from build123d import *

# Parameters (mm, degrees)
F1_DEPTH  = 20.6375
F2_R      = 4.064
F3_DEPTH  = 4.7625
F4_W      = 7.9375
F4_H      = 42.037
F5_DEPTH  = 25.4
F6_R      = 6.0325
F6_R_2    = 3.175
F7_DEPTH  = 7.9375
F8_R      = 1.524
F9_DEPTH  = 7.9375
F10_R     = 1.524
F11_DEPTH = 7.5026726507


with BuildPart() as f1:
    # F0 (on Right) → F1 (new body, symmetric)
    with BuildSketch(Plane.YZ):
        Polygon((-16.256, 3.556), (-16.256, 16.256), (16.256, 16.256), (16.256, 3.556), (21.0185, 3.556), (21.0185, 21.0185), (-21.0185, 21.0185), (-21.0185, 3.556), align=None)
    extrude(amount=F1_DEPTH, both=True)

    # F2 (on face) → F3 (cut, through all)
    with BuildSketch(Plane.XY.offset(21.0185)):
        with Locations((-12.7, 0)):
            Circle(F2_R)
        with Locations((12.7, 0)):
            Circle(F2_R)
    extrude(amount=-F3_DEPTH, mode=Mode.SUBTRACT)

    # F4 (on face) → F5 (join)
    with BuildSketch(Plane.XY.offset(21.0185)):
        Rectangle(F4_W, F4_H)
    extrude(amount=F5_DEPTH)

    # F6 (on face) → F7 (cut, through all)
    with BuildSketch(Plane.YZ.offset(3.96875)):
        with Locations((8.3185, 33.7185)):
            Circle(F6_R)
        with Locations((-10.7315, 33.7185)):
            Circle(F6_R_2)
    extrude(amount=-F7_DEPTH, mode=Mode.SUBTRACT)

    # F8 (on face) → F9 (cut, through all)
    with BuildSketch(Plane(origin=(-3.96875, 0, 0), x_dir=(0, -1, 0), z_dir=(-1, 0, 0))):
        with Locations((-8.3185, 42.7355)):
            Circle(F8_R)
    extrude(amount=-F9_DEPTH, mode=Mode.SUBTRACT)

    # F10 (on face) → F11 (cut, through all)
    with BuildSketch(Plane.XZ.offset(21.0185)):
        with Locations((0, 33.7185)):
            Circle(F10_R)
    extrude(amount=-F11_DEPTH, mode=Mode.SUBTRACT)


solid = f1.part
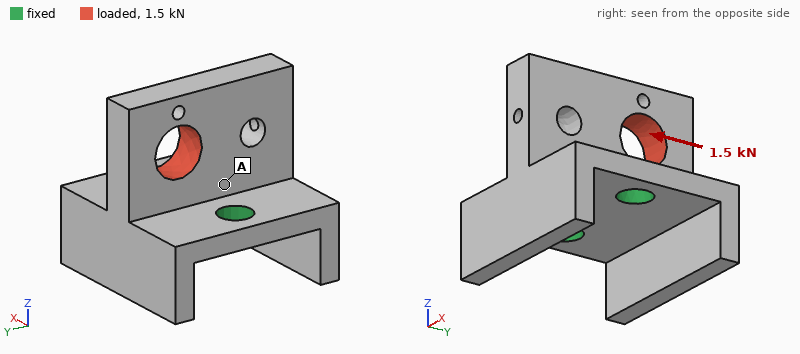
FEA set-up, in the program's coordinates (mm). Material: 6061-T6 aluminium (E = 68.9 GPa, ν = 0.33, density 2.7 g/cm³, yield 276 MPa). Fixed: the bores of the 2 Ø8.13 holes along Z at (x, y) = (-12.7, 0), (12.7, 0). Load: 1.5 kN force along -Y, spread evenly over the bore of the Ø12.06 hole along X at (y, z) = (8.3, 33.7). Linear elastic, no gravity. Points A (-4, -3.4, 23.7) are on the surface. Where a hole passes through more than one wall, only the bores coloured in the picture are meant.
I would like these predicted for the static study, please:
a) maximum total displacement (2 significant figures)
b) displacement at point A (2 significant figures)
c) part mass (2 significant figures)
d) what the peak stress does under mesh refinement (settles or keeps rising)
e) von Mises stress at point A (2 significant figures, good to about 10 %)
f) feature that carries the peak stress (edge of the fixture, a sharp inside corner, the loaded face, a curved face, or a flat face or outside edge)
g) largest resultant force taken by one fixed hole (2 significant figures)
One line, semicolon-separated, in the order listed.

60 µm; 10 µm; 54 g; keeps rising; 14 MPa; edge of the fixture; 750 N
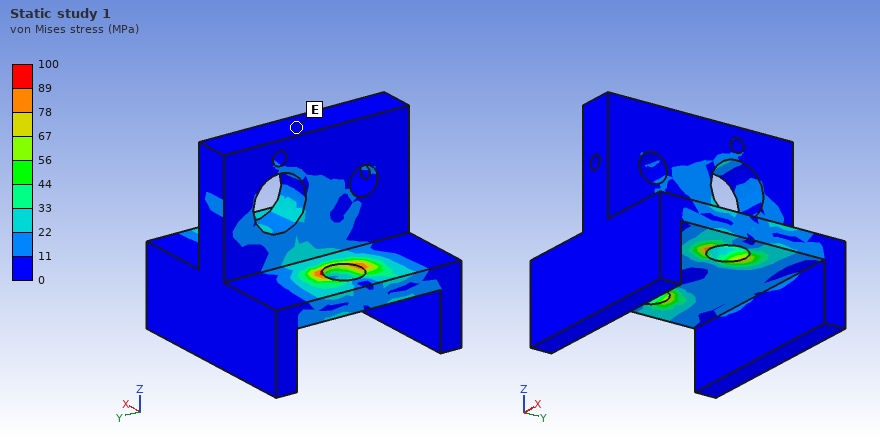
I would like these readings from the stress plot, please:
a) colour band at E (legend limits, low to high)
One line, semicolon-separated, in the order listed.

0 to 11 MPa
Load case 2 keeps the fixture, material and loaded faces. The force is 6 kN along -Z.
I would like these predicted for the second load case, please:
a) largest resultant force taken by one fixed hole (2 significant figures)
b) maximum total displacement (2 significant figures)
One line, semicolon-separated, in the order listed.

3.1 kN; 0.13 mm
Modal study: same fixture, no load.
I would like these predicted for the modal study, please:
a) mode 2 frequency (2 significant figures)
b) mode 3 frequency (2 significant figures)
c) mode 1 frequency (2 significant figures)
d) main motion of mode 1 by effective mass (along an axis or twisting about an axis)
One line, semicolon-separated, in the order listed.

6500 Hz; 8900 Hz; 4500 Hz; twisting about X
